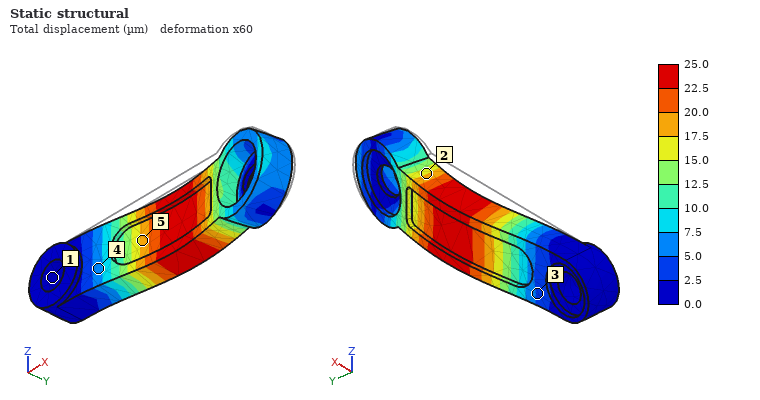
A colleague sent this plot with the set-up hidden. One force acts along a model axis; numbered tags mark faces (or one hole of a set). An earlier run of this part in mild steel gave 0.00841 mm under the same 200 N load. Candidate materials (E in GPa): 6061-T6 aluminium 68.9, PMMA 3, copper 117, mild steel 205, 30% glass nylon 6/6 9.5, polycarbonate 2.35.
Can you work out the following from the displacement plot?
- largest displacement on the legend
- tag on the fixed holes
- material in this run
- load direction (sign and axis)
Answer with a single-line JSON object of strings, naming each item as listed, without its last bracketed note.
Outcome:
{"largest displacement on the legend": "25.0 µm", "tag on the fixed holes": "1", "material in this run": "6061-T6 aluminium", "load direction": "+Y"}
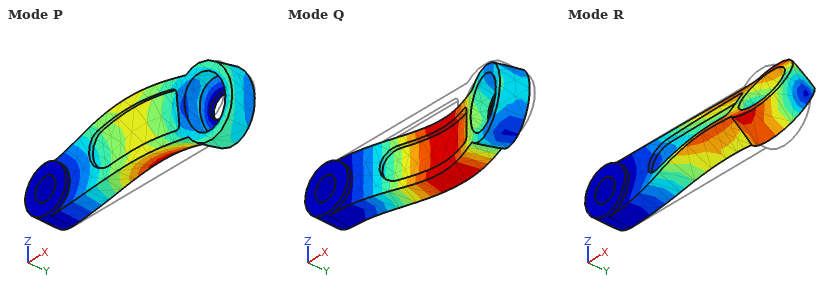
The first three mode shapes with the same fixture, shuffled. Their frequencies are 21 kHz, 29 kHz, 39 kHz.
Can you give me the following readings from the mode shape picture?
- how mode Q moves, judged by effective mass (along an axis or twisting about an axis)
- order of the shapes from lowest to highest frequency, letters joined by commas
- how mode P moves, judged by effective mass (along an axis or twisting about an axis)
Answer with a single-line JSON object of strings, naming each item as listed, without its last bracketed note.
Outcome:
{"how mode Q moves, judged by effective mass": "along Y", "order of the shapes from lowest to highest frequency, letters joined by commas": "Q, R, P", "how mode P moves, judged by effective mass": "along Z"}
